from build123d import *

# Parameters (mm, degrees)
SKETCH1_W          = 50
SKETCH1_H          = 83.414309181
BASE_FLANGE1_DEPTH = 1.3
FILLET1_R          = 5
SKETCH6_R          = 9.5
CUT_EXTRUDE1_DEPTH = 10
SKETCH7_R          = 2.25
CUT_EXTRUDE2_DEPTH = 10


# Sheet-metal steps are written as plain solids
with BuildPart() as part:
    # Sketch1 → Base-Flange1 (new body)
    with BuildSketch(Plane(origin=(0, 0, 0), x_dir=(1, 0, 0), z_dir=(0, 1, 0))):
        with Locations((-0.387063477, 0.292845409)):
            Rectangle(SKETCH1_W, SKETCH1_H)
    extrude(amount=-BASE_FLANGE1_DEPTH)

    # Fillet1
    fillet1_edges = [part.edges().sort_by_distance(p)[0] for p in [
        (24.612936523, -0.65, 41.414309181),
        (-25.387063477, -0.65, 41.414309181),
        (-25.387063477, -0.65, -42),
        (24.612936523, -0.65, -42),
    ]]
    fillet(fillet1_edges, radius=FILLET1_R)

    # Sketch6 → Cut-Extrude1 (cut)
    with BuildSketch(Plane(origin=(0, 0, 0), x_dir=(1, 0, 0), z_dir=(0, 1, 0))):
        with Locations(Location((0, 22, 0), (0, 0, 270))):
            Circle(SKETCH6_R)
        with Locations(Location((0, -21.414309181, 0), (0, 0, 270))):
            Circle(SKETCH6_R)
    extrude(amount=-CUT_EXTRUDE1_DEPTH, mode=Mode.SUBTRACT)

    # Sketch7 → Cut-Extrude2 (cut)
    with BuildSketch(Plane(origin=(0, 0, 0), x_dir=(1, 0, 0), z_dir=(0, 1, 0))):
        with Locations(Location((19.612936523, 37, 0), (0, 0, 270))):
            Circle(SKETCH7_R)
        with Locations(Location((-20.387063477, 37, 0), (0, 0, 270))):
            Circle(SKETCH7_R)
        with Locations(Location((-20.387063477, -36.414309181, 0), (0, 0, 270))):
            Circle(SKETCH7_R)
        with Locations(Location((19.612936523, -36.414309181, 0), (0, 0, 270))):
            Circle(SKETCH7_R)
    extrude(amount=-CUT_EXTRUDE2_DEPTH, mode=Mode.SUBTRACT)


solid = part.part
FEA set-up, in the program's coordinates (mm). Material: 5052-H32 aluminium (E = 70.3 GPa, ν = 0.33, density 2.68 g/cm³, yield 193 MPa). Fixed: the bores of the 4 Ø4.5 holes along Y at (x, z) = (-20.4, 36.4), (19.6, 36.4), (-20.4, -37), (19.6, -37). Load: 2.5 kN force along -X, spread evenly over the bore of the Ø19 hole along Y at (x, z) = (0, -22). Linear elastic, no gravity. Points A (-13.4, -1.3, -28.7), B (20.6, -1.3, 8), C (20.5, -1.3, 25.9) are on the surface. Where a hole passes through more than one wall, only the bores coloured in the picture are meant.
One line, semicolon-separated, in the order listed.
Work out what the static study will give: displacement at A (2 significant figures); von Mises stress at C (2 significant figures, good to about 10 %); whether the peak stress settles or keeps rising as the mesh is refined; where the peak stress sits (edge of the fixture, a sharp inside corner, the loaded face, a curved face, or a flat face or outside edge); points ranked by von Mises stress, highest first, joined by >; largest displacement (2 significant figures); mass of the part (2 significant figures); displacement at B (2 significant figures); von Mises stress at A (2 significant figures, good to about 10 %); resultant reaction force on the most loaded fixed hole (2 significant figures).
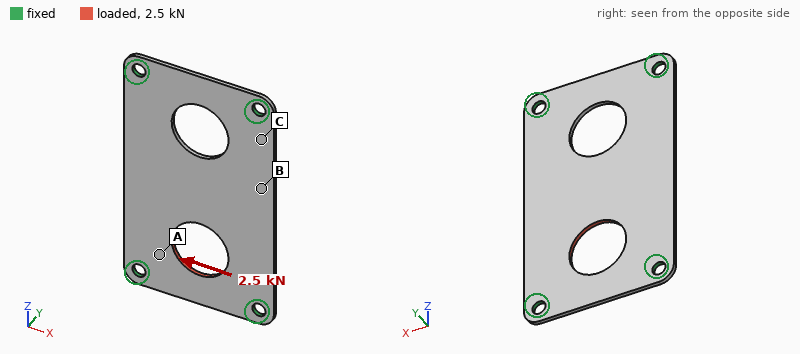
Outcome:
16 µm; 28 MPa; keeps rising; edge of the fixture; A > C > B; 42 µm; 12 g; 29 µm; 57 MPa; 1.0 kN
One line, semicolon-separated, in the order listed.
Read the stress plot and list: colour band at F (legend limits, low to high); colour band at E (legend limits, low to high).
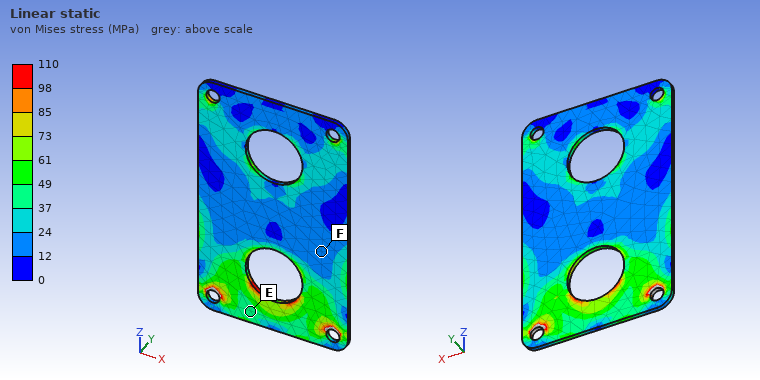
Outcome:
12 to 24 MPa; 37 to 49 MPa
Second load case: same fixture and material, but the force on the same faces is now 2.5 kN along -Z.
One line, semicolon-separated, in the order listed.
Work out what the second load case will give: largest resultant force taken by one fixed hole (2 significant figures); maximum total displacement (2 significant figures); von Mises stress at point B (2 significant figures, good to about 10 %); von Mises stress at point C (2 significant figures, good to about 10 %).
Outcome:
920 N; 28 µm; 14 MPa; 22 MPa
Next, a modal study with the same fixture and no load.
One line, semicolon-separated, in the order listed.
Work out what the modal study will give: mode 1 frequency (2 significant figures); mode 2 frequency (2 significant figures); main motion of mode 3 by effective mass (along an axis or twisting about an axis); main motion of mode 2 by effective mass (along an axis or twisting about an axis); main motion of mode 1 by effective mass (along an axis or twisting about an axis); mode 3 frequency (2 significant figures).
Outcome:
1200 Hz; 1800 Hz; twisting about X; twisting about Z; along Y; 3400 Hz
